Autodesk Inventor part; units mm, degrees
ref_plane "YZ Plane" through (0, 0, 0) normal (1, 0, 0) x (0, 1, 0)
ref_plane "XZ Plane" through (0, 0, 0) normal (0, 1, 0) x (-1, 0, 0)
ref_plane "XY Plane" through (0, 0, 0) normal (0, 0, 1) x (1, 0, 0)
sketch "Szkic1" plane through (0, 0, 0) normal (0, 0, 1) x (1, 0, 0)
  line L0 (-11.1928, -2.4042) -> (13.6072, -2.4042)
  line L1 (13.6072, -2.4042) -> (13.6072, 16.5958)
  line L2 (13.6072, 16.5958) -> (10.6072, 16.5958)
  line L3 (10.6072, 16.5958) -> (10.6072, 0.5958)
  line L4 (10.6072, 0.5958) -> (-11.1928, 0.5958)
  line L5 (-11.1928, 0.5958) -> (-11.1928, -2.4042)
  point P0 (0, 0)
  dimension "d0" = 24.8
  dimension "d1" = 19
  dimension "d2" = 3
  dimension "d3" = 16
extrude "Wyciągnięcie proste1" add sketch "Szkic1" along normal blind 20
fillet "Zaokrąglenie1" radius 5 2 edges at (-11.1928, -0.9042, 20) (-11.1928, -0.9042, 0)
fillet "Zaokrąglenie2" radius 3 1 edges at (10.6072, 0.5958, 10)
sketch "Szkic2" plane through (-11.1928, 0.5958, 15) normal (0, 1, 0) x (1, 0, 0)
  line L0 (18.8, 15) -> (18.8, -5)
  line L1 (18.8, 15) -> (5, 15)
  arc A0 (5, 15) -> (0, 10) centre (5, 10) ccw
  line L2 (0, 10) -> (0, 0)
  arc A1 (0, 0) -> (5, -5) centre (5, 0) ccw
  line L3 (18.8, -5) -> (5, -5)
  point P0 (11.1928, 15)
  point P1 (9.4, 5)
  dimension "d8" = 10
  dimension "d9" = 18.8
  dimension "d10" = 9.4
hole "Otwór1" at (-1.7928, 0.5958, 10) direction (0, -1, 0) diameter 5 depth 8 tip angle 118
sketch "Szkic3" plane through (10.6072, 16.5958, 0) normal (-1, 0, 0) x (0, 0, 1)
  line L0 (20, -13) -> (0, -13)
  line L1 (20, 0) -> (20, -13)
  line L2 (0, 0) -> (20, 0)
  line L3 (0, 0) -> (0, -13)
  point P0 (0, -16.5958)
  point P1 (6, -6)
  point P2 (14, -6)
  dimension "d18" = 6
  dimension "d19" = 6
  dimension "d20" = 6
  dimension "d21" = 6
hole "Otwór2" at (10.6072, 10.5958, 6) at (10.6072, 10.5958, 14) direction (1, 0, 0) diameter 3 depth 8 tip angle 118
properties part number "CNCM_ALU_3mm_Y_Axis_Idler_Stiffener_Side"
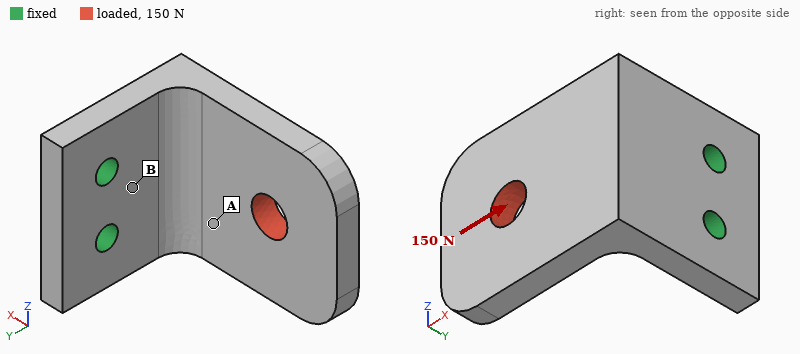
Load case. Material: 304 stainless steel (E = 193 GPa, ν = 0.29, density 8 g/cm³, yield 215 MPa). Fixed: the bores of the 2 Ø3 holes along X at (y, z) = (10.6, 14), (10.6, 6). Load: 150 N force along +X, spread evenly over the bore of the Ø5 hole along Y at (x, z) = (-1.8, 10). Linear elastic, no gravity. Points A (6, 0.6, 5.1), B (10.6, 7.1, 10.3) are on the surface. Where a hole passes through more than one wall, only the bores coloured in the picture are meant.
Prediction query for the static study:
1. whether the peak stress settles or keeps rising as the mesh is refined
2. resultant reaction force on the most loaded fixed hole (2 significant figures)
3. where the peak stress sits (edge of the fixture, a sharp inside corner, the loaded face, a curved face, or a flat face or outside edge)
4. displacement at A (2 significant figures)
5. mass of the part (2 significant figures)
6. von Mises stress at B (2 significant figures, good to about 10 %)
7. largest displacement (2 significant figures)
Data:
keeps rising
75 N
edge of the fixture
8.8 µm
19 g
35 MPa
25 µm
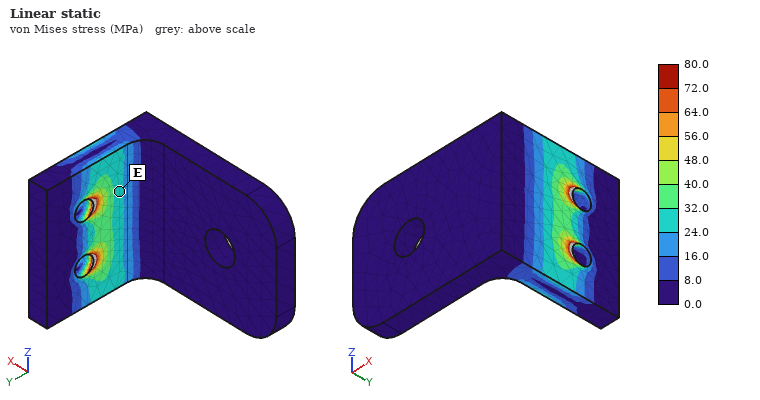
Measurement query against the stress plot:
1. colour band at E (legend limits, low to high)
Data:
24.0 to 32.0 MPa
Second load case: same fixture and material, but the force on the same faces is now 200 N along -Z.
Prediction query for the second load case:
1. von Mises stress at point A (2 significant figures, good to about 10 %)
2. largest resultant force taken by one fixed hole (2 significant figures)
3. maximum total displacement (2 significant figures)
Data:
21 MPa
320 N
28 µm
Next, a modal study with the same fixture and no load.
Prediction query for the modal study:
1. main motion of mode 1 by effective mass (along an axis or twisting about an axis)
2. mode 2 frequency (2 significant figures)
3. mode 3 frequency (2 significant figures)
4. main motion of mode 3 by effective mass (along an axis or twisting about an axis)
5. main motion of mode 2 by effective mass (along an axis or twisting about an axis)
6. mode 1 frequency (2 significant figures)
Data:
along Y
5300 Hz
9700 Hz
along X
along Z
2900 Hz
